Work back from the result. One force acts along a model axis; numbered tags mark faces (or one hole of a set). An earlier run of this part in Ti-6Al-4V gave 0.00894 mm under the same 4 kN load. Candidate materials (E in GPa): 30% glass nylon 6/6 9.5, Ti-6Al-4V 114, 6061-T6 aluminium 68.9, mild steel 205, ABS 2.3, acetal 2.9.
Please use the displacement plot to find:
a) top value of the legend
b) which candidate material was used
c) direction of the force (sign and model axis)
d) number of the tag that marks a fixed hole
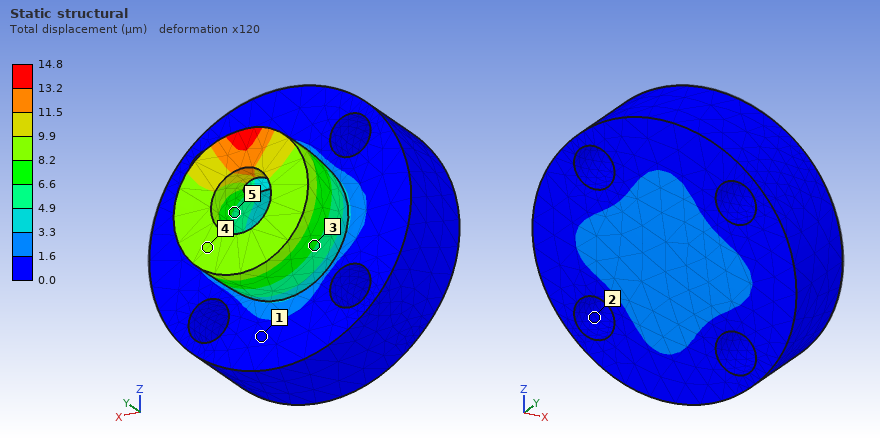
14.8 µm
6061-T6 aluminium
-Y
2
